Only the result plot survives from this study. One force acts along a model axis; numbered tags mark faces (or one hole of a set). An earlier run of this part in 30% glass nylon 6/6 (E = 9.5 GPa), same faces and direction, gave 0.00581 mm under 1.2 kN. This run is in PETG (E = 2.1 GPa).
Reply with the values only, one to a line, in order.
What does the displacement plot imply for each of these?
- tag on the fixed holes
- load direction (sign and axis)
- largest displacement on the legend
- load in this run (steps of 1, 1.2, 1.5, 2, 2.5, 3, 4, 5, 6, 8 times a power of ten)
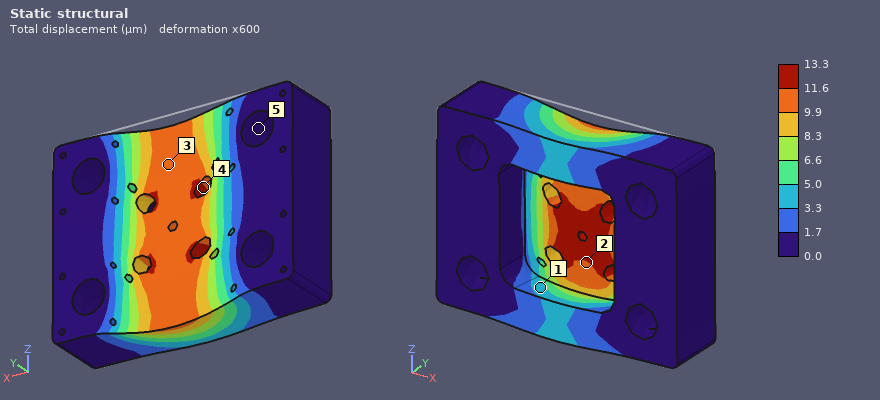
5
-Z
13.3 µm
600 N
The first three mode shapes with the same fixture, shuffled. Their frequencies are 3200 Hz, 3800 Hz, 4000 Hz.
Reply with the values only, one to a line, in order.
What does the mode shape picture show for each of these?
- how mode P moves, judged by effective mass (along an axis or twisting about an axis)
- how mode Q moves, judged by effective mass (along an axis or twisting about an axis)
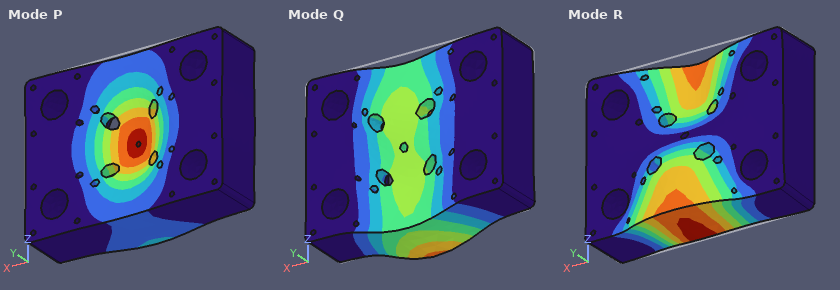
along Y
along Z
